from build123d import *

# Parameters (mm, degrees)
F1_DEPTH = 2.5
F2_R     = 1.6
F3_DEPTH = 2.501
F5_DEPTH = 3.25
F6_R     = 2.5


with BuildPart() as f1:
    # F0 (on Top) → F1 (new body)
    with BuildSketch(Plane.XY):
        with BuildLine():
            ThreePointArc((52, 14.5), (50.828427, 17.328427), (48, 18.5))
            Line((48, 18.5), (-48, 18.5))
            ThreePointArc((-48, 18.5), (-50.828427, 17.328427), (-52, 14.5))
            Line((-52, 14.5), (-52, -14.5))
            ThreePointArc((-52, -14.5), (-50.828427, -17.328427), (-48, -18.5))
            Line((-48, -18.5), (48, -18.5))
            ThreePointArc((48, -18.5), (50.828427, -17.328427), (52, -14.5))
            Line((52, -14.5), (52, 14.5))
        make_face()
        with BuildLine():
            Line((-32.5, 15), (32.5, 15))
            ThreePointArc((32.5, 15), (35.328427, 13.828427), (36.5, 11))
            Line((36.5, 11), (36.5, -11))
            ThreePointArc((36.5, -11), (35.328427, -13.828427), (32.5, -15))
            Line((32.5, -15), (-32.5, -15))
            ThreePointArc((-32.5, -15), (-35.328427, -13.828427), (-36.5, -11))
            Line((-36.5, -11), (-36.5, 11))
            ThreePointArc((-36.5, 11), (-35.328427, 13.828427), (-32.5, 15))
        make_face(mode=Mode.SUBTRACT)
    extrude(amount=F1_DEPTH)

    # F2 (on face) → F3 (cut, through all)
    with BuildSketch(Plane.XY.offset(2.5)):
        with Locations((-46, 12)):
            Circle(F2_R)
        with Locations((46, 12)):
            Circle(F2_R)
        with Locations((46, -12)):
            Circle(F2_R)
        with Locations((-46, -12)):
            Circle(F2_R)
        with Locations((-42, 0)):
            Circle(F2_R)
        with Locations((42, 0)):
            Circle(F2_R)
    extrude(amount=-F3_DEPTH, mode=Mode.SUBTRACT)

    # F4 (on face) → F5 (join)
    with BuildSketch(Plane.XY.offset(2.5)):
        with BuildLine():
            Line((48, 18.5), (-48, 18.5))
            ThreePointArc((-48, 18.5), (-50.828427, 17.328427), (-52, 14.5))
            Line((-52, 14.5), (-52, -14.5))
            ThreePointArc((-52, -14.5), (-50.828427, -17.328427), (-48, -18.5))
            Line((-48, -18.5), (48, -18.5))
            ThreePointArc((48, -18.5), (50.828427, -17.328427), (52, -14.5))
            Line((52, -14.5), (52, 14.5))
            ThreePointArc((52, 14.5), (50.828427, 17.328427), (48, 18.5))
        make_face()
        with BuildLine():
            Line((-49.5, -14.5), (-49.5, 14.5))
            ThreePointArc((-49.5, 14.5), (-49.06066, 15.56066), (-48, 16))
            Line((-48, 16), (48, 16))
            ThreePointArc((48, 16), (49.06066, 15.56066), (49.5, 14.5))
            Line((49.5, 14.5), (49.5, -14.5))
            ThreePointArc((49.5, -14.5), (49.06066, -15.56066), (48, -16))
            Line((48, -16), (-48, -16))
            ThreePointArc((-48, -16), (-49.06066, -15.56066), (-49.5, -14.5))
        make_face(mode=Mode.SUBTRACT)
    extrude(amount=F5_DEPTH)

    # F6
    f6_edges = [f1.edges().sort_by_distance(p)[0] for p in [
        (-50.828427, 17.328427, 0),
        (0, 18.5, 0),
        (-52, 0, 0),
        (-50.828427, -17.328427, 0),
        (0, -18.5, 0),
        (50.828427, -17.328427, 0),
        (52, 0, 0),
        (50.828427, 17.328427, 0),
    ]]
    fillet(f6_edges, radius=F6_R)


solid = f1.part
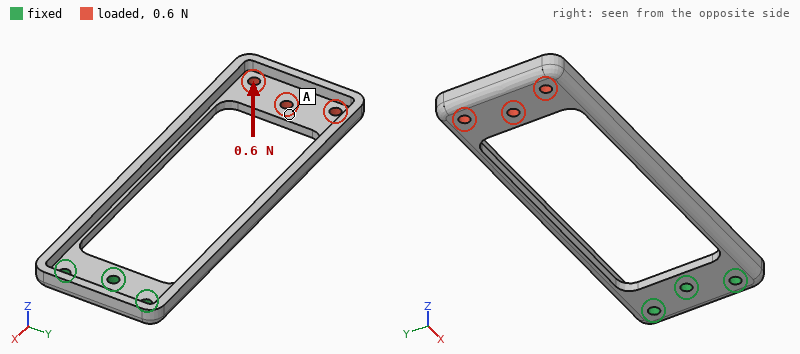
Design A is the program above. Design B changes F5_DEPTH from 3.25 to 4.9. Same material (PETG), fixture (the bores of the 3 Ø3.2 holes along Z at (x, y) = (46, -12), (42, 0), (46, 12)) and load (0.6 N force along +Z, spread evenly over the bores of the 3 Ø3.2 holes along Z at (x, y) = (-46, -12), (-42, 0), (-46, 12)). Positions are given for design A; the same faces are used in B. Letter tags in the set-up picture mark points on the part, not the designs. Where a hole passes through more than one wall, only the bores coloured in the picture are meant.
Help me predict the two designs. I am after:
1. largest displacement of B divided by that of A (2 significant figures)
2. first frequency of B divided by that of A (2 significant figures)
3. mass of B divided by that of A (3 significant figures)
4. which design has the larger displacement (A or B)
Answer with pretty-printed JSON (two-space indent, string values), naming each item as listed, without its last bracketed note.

{
  "largest displacement of B divided by that of A": "0.53",
  "first frequency of B divided by that of A": "1.3",
  "mass of B divided by that of A": "1.19",
  "which design has the larger displacement": "A"
}
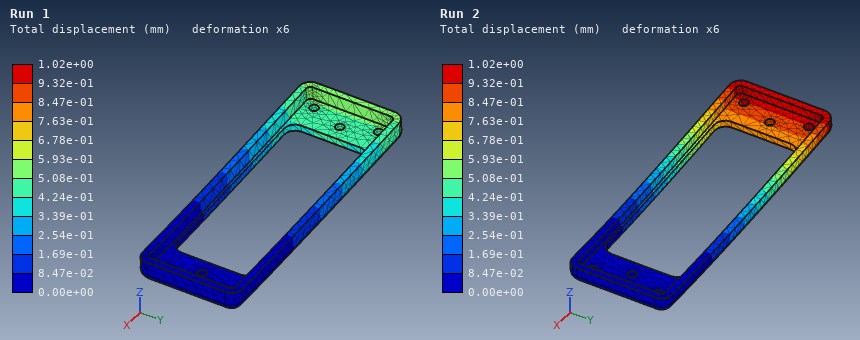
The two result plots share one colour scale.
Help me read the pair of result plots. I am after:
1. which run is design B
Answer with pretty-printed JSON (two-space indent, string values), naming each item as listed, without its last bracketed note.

{
  "which run is design B": "Run 1"
}
